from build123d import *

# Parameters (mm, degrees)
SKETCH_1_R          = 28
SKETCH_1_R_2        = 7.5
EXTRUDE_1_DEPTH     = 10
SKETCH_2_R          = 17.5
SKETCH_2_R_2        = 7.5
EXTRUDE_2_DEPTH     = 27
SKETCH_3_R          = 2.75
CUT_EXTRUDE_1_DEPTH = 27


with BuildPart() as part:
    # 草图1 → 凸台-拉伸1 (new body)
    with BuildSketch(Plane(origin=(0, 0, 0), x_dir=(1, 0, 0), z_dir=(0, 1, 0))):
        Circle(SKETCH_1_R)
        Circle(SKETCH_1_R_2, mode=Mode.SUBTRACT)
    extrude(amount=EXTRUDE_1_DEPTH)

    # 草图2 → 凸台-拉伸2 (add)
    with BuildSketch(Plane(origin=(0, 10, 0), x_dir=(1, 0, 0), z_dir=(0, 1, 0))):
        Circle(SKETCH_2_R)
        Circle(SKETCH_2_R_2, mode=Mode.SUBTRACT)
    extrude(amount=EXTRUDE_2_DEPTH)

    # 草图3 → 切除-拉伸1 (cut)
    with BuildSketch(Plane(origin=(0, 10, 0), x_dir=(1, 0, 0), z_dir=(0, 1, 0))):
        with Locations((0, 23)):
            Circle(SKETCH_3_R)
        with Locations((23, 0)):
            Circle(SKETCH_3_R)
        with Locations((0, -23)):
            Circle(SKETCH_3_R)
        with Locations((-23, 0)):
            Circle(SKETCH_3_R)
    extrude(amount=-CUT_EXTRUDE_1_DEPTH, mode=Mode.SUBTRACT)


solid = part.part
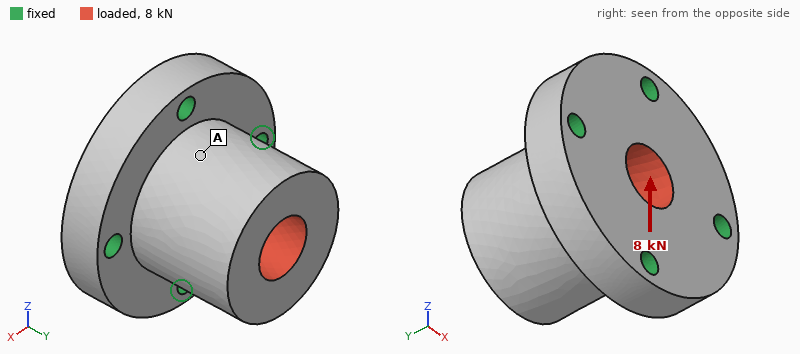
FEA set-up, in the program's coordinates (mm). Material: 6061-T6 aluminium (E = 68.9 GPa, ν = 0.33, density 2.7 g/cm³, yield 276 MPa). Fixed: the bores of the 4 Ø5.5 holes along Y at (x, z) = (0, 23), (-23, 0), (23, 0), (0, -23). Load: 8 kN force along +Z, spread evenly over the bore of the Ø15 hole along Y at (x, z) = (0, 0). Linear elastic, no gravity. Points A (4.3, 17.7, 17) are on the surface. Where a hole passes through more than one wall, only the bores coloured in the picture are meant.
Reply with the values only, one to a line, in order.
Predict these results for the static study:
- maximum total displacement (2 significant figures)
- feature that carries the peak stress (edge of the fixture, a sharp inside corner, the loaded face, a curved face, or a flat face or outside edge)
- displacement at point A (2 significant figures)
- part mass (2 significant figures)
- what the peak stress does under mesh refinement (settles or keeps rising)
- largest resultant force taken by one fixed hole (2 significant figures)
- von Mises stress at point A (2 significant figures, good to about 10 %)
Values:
21 µm
edge of the fixture
11 µm
120 g
keeps rising
3.5 kN
9.9 MPa
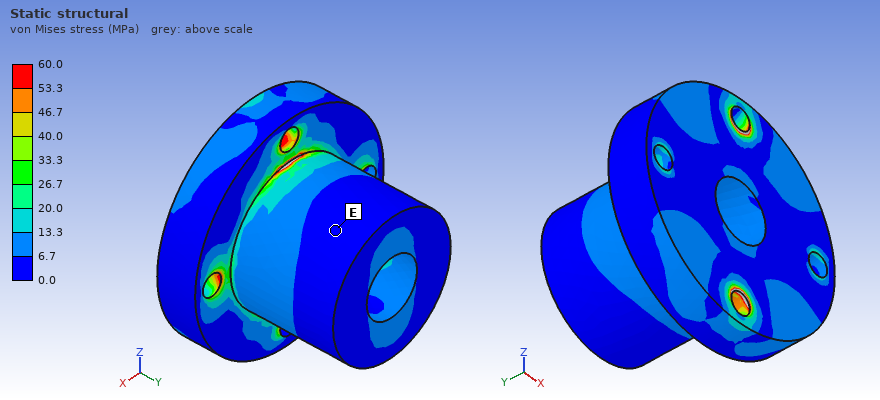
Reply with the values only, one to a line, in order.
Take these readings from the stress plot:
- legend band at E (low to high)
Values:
0.0 to 6.7 MPa
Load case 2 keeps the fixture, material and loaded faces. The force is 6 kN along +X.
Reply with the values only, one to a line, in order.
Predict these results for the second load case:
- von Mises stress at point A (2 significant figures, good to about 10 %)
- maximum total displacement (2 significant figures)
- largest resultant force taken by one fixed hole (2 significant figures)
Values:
7.5 MPa
16 µm
2.6 kN
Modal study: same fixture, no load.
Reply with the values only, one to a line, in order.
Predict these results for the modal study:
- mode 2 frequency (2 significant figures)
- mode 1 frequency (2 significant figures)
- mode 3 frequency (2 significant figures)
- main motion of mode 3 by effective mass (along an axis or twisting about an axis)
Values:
13 kHz
13 kHz
20 kHz
along Y
